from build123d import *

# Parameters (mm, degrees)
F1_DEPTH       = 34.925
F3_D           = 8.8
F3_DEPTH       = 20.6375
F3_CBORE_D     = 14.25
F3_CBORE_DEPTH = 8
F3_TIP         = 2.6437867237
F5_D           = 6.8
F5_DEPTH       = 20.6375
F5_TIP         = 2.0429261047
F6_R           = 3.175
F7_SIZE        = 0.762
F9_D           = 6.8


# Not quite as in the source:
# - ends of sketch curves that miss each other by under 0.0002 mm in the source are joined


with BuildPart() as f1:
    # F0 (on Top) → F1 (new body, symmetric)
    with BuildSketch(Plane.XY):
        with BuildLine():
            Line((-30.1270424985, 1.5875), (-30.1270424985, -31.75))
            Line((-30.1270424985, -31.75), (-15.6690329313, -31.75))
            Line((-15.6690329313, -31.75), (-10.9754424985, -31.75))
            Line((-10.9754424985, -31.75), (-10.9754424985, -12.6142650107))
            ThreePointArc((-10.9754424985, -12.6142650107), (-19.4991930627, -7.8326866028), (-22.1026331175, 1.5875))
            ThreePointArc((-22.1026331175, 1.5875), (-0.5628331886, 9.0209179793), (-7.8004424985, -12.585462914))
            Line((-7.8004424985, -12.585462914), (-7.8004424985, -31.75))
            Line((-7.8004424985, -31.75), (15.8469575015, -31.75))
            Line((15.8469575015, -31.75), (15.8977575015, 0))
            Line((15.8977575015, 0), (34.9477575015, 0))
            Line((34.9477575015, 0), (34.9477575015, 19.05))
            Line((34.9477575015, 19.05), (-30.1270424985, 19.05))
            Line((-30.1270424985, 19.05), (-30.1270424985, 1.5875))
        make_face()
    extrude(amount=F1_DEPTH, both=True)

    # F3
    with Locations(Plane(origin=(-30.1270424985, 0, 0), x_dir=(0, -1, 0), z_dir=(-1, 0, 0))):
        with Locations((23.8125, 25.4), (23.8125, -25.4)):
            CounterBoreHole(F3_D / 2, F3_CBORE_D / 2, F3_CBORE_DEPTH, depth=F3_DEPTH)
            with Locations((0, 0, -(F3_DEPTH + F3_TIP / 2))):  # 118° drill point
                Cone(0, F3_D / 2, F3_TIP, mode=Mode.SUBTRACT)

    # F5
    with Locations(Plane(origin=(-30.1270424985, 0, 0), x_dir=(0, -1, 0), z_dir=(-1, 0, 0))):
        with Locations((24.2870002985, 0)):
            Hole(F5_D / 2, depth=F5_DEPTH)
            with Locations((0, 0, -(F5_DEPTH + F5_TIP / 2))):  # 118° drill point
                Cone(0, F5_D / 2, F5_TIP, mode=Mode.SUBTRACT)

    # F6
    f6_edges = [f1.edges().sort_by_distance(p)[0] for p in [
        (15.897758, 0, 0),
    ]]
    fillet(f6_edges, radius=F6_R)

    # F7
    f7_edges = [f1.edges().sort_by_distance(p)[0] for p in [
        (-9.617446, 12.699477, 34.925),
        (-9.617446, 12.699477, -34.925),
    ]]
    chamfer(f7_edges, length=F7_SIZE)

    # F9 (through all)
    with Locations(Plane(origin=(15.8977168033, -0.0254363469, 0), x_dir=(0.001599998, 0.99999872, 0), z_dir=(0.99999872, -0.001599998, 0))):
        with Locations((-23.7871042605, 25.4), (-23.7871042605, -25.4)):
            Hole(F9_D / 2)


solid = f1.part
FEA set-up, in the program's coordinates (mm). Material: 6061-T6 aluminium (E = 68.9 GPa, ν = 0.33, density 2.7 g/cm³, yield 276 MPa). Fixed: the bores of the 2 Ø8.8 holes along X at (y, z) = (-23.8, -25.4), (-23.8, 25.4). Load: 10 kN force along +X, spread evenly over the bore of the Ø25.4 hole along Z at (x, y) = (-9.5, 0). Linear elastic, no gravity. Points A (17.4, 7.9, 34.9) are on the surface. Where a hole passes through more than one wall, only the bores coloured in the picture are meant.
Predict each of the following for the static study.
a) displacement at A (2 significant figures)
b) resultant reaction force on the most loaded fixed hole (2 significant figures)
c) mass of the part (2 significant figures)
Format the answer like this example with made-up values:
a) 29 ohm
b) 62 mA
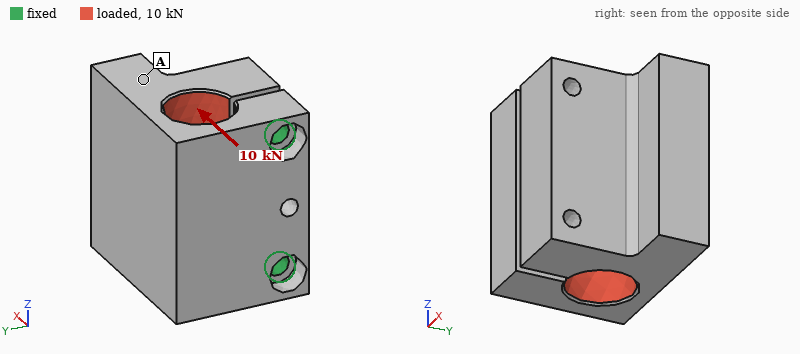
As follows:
a) 0.23 mm
b) 5.1 kN
c) 390 g
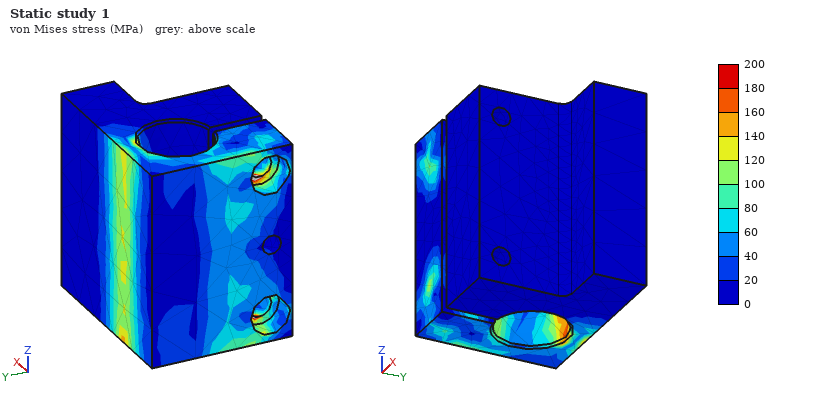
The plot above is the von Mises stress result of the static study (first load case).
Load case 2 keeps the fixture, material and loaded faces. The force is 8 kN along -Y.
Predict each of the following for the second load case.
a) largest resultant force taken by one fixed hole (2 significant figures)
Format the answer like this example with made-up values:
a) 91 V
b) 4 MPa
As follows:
a) 4.1 kN
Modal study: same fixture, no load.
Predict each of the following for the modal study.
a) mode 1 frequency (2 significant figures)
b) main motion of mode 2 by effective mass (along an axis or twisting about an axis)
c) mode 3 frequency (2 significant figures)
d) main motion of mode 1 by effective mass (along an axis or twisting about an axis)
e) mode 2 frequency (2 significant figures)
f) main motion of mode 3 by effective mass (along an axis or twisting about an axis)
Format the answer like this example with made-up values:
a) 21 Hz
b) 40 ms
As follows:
a) 600 Hz
b) along Z
c) 1500 Hz
d) along Y
e) 1100 Hz
f) along X
